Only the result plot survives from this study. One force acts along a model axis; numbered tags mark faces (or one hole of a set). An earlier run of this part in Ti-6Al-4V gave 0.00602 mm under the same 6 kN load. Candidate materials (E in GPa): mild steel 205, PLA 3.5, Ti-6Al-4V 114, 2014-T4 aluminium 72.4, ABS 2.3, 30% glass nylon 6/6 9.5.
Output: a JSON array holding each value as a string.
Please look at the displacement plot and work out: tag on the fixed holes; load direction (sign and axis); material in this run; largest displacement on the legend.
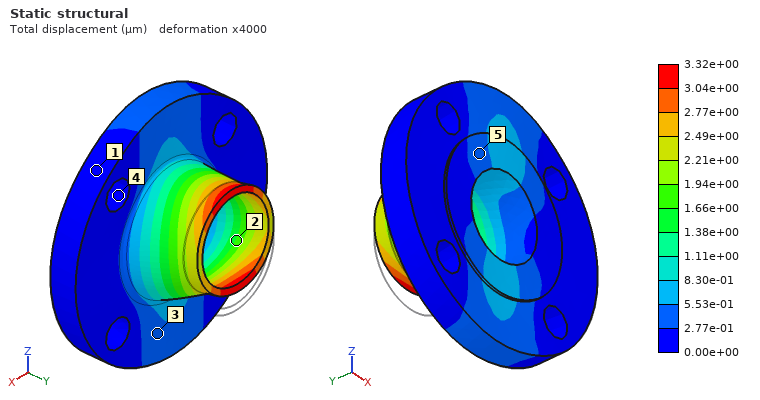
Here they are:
["4", "+Z", "mild steel", "3.32e+00 µm"]
